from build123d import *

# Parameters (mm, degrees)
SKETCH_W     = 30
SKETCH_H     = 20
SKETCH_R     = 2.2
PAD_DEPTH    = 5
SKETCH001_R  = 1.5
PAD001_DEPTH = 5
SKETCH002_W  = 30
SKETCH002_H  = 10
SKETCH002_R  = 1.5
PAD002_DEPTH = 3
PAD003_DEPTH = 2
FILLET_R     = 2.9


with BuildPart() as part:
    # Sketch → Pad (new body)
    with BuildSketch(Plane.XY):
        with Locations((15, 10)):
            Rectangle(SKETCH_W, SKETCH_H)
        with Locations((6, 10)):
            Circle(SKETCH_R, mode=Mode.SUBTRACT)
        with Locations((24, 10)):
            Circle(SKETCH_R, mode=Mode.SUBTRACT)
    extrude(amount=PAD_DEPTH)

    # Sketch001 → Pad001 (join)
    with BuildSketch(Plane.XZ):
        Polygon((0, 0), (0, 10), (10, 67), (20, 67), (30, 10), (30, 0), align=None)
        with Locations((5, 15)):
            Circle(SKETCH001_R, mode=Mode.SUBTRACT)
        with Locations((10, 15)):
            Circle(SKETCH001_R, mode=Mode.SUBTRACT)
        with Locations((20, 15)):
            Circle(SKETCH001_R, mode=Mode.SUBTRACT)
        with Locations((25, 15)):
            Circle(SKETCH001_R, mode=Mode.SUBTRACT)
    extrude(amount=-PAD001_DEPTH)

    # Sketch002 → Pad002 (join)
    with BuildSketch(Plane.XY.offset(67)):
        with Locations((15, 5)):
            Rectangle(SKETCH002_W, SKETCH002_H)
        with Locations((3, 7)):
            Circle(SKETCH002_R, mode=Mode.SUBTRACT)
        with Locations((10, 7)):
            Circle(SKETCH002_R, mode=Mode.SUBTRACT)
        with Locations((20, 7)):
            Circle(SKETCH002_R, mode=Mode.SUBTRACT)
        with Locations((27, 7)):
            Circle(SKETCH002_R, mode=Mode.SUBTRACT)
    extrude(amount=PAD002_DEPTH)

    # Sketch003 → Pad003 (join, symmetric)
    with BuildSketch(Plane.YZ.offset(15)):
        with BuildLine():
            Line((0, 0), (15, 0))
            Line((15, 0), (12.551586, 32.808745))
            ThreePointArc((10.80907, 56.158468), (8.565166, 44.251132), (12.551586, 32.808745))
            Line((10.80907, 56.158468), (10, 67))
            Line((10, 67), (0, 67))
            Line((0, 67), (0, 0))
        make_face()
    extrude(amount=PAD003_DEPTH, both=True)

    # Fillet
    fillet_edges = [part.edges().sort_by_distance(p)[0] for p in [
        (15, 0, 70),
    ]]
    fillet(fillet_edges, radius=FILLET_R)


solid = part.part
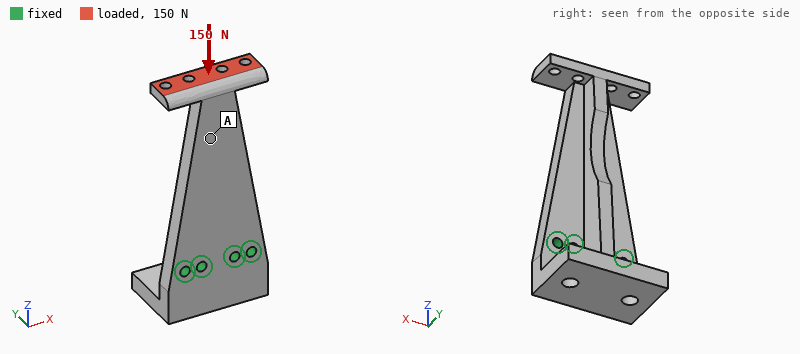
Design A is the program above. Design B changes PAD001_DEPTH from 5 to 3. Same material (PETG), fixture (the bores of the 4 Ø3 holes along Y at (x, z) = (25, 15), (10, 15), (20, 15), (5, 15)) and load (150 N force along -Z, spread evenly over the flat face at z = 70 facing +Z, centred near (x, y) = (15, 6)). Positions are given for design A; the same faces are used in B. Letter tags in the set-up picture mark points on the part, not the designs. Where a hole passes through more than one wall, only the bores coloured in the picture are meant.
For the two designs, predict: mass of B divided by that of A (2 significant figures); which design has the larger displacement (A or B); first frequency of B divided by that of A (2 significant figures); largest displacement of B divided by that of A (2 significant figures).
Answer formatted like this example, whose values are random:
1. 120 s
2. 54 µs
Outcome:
1. 0.82
2. B
3. 0.78
4. 1.4
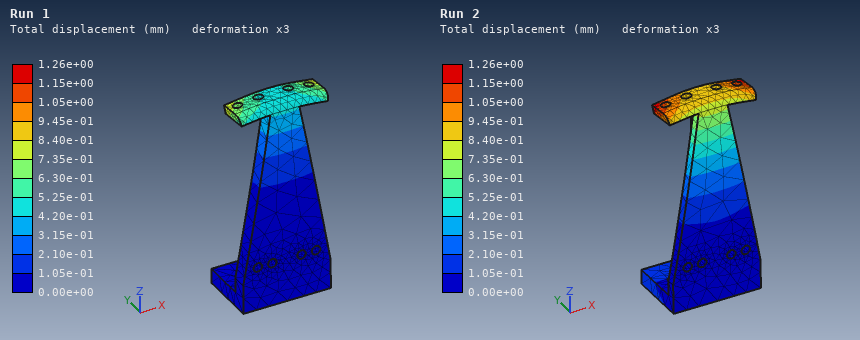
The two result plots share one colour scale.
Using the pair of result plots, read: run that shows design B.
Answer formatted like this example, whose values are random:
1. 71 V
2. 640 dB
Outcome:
1. Run 2
